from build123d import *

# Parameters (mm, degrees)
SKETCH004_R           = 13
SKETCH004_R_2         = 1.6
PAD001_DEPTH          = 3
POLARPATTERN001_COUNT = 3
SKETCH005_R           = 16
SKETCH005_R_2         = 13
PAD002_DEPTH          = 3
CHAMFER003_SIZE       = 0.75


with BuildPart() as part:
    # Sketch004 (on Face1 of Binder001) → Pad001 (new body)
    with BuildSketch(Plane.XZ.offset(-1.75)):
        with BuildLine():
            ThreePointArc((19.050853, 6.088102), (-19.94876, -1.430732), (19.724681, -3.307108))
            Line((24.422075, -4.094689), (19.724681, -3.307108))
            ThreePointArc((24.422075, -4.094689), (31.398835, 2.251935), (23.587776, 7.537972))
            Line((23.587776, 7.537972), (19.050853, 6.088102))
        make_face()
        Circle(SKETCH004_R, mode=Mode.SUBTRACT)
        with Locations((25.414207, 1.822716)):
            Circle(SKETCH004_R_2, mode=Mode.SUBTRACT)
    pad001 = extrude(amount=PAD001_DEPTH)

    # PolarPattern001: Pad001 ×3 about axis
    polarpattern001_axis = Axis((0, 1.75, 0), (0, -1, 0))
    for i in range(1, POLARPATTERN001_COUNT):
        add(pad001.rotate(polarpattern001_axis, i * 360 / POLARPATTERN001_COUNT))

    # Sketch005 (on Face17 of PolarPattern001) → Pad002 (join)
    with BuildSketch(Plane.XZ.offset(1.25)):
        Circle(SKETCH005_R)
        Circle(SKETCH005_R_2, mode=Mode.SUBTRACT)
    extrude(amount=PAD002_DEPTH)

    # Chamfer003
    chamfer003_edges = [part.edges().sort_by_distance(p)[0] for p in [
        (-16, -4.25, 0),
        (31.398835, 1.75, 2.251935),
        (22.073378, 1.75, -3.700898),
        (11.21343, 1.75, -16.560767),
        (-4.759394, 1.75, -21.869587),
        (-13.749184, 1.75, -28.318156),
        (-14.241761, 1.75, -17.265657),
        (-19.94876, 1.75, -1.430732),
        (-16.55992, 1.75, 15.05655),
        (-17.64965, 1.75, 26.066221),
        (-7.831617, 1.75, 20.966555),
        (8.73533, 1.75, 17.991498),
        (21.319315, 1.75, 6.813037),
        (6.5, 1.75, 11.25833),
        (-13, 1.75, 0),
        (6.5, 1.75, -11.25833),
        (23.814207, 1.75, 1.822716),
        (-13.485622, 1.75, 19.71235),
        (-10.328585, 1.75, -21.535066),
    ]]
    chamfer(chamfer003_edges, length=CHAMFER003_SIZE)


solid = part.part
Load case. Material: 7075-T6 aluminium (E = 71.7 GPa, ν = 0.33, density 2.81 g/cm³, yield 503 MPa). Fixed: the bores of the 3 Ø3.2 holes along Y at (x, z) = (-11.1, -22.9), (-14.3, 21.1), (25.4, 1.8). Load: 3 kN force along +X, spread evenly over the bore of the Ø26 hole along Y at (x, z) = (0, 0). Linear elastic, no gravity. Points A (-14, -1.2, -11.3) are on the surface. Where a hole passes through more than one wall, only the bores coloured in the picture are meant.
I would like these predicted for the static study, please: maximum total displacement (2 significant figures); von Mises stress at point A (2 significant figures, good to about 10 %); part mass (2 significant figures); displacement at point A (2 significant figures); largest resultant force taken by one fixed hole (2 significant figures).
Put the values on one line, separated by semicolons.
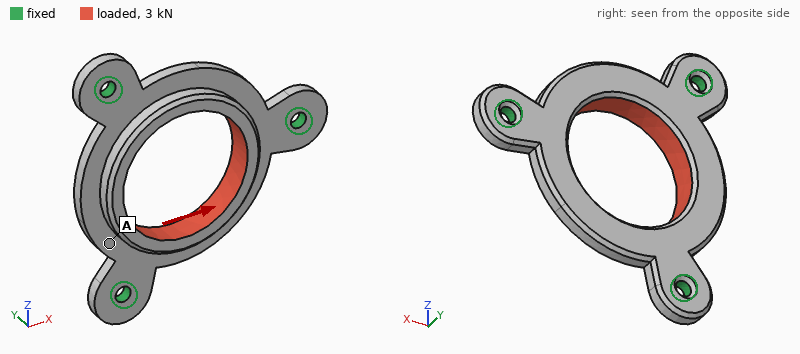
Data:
61 µm; 42 MPa; 11 g; 39 µm; 1.1 kN
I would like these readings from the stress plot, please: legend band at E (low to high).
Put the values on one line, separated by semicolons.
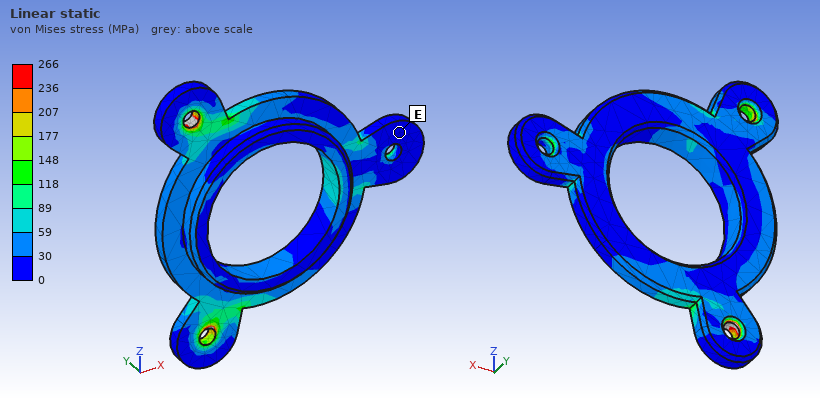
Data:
0 to 30 MPa
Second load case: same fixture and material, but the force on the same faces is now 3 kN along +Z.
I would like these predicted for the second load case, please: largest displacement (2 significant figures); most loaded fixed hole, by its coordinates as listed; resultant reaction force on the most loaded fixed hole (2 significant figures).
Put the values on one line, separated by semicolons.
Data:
56 µm; (25.4, 1.8); 1.1 kN
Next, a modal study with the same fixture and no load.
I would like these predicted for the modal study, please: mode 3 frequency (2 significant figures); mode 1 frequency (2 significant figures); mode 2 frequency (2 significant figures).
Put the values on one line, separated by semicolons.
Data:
8600 Hz; 8500 Hz; 8600 Hz
